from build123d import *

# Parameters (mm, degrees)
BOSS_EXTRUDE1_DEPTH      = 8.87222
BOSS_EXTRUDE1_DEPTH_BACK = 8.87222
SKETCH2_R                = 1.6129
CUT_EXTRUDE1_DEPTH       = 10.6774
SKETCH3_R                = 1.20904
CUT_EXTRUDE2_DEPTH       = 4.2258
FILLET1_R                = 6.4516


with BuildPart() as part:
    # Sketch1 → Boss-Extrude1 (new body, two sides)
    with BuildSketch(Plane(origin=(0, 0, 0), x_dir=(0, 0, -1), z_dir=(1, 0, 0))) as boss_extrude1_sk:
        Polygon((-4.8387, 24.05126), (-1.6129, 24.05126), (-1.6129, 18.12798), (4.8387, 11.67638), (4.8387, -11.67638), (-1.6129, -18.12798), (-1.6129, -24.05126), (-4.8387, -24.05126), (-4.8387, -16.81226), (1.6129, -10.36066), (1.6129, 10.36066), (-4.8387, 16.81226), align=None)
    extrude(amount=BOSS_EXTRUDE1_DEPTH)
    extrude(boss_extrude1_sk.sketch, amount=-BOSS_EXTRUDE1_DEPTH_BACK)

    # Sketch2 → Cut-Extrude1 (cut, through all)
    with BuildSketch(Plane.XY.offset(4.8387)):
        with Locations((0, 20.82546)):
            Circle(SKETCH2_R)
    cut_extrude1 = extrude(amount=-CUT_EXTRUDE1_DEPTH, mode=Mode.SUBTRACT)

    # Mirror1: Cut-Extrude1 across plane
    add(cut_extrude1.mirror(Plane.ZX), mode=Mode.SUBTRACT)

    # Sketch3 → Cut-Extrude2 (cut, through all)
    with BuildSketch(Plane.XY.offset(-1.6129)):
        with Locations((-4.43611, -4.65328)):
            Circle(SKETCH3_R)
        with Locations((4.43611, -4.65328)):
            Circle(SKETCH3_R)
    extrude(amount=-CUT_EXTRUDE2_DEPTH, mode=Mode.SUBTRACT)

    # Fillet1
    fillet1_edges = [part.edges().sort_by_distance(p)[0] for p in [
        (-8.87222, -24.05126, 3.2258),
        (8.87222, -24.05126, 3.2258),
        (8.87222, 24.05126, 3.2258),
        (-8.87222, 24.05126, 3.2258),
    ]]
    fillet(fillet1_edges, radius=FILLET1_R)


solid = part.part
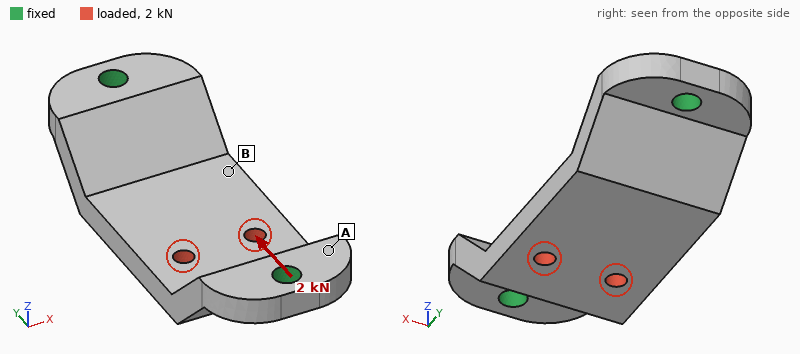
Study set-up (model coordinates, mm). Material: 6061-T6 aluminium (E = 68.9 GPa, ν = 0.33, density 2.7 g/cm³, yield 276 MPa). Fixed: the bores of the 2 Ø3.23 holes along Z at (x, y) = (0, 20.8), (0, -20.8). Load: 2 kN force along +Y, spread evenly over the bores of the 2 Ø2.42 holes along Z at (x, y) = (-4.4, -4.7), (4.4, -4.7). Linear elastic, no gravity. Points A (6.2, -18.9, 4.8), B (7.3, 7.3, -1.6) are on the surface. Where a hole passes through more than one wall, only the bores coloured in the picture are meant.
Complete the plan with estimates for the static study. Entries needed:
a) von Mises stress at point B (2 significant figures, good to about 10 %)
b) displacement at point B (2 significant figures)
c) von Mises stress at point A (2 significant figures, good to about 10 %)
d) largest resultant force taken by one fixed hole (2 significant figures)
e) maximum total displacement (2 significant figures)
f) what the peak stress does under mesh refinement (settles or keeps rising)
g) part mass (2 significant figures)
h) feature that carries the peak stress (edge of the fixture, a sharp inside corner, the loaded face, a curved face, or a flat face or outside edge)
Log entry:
70 MPa
29 µm
30 MPa
1.0 kN
33 µm
keeps rising
7.7 g
a sharp inside corner
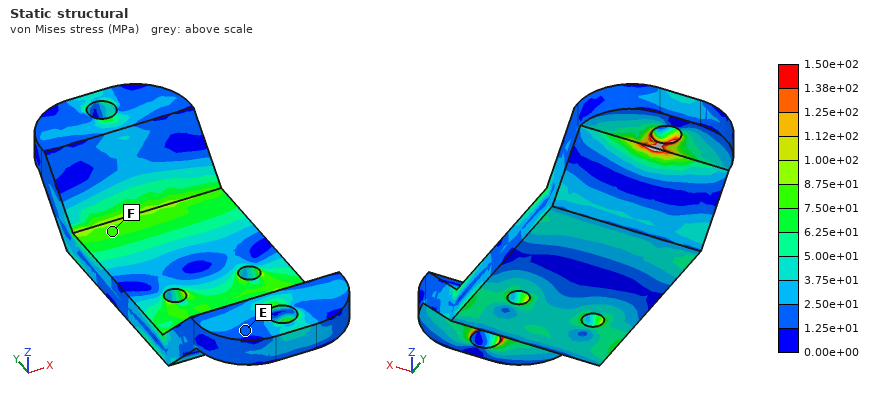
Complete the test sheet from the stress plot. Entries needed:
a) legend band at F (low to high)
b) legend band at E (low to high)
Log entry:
7.50e+01 to 8.75e+01 MPa
1.25e+01 to 2.50e+01 MPa
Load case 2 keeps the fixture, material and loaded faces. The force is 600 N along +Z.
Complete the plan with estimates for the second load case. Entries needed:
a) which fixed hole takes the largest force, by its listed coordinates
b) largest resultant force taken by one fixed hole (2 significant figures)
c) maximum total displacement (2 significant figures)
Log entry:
(0, -20.8)
640 N
26 µm
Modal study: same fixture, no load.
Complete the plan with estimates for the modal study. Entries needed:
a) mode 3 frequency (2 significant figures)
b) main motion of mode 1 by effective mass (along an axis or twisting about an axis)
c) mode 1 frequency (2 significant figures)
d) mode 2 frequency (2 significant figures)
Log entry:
17 kHz
along X
10000 Hz
17 kHz
